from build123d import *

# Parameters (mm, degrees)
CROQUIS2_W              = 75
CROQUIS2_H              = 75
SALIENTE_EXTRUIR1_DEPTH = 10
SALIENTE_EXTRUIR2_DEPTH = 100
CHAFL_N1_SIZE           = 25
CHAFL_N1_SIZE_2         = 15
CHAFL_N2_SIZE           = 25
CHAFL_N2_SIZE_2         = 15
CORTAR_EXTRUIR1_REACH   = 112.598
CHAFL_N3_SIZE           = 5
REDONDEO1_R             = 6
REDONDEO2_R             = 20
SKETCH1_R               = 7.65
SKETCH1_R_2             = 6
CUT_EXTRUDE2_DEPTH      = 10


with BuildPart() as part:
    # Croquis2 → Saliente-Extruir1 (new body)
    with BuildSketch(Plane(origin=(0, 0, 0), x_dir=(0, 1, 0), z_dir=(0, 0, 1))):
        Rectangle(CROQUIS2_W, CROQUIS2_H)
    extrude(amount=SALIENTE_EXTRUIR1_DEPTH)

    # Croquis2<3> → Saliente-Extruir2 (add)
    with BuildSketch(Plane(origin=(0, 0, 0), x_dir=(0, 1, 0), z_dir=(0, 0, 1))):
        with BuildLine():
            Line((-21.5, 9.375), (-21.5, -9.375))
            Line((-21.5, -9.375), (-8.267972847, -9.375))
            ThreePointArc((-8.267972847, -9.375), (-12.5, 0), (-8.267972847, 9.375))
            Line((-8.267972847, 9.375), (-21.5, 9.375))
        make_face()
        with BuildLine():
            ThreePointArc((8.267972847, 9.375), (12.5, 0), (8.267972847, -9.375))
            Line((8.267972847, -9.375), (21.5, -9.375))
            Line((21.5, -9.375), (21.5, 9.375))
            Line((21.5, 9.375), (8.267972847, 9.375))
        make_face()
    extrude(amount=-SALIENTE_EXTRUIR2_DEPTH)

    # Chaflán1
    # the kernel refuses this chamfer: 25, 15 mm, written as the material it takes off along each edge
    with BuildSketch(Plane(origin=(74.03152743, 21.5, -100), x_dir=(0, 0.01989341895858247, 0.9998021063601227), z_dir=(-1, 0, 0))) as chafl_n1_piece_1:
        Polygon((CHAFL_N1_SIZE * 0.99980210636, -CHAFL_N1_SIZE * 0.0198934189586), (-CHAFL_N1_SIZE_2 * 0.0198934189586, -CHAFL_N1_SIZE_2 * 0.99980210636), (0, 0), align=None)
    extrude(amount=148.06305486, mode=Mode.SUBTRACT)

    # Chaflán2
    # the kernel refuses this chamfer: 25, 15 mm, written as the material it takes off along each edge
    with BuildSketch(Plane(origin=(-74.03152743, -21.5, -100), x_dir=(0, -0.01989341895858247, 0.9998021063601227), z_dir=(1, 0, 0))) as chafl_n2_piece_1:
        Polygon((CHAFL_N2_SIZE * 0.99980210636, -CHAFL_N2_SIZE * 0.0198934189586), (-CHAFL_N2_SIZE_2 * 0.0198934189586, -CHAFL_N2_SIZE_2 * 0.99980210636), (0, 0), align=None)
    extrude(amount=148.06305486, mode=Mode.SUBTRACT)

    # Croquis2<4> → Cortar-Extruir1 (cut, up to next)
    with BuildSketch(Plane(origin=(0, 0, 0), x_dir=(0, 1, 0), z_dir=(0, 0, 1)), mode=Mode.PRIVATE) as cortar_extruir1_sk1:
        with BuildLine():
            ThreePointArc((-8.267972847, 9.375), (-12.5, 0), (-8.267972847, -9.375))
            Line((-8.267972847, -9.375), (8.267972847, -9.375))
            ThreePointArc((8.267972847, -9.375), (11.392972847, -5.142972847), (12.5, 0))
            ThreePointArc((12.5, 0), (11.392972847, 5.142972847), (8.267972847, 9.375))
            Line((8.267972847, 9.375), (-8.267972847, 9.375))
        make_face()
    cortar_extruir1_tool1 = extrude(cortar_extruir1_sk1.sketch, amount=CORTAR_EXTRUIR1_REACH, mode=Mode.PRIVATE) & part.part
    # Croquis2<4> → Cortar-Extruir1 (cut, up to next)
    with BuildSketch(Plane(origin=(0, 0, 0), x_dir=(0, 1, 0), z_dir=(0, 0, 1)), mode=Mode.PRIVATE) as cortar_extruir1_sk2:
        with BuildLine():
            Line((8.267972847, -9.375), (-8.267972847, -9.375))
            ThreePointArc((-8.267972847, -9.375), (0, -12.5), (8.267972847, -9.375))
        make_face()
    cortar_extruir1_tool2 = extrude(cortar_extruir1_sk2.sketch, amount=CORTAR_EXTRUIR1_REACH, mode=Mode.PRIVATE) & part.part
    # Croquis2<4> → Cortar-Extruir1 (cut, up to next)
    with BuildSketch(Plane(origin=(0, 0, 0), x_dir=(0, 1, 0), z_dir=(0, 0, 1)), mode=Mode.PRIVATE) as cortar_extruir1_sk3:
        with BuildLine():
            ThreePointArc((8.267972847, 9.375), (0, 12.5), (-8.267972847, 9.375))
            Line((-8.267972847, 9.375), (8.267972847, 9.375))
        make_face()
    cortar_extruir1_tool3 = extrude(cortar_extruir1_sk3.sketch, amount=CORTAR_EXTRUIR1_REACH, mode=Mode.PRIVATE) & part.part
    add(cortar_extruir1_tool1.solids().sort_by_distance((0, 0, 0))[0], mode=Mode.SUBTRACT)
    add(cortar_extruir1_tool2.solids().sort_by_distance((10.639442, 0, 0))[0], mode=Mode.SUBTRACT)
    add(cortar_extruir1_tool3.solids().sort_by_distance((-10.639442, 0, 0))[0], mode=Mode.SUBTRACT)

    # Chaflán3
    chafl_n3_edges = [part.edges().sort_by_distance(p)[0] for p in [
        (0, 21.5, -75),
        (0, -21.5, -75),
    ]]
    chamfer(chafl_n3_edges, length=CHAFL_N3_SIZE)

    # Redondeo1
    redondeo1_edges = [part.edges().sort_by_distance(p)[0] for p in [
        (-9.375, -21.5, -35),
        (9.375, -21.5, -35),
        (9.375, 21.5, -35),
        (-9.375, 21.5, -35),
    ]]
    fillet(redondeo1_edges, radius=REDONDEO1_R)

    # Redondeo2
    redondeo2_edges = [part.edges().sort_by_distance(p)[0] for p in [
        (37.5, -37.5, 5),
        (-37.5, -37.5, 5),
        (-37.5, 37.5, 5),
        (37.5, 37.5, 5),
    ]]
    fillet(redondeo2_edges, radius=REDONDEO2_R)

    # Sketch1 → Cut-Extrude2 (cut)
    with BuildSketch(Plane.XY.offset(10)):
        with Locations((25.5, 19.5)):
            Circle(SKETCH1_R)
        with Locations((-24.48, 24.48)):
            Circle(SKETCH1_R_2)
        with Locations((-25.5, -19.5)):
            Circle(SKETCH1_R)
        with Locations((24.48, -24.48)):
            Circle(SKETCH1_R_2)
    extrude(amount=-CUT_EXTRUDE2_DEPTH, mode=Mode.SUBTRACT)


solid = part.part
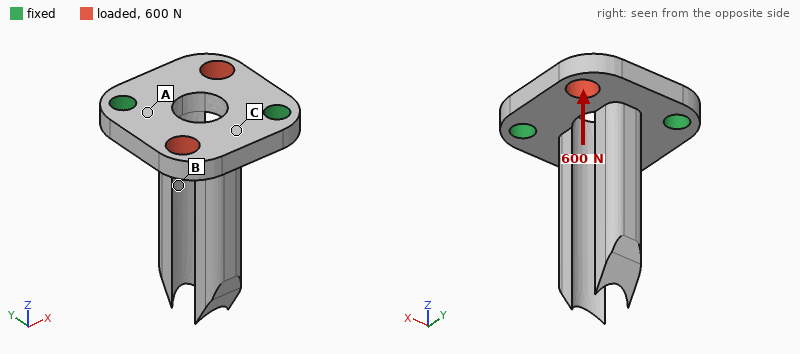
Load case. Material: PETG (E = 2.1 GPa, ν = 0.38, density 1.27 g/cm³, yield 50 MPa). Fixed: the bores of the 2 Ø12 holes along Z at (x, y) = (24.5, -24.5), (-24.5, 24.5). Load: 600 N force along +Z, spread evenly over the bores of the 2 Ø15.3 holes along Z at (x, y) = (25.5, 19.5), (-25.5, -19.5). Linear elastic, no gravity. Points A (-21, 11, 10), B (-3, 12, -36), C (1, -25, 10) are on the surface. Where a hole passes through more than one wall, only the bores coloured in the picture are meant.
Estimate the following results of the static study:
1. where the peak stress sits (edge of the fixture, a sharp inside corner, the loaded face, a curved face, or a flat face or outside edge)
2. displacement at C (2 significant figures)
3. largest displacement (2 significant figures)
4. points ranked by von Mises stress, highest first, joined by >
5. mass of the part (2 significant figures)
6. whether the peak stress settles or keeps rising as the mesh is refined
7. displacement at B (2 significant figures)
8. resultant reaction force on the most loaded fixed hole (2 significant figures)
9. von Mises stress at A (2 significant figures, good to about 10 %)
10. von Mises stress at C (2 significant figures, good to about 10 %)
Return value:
a sharp inside corner
0.14 mm
0.85 mm
A > C > B
91 g
keeps rising
0.35 mm
300 N
7.3 MPa
4.6 MPa
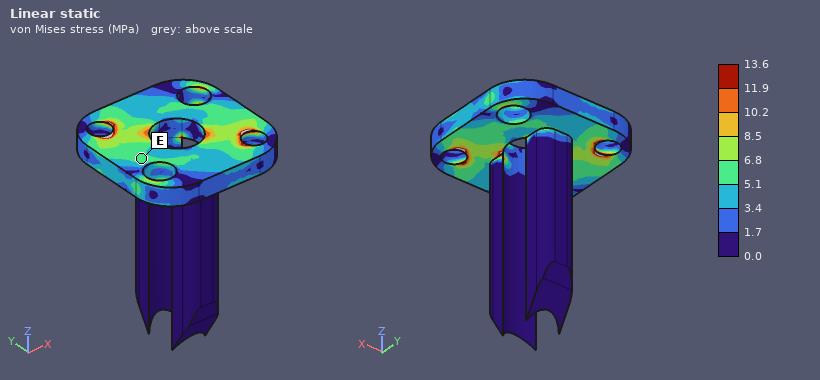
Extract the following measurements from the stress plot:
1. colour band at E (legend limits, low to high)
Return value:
5.1 to 6.8 MPa
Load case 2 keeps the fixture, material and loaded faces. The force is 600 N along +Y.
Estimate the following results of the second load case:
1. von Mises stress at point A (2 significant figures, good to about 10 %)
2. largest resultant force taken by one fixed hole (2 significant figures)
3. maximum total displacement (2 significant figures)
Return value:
1.4 MPa
300 N
42 µm
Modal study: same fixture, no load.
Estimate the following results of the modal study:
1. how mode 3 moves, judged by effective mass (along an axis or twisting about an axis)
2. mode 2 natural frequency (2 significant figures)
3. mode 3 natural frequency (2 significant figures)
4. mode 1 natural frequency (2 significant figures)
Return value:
along X
260 Hz
370 Hz
250 Hz
